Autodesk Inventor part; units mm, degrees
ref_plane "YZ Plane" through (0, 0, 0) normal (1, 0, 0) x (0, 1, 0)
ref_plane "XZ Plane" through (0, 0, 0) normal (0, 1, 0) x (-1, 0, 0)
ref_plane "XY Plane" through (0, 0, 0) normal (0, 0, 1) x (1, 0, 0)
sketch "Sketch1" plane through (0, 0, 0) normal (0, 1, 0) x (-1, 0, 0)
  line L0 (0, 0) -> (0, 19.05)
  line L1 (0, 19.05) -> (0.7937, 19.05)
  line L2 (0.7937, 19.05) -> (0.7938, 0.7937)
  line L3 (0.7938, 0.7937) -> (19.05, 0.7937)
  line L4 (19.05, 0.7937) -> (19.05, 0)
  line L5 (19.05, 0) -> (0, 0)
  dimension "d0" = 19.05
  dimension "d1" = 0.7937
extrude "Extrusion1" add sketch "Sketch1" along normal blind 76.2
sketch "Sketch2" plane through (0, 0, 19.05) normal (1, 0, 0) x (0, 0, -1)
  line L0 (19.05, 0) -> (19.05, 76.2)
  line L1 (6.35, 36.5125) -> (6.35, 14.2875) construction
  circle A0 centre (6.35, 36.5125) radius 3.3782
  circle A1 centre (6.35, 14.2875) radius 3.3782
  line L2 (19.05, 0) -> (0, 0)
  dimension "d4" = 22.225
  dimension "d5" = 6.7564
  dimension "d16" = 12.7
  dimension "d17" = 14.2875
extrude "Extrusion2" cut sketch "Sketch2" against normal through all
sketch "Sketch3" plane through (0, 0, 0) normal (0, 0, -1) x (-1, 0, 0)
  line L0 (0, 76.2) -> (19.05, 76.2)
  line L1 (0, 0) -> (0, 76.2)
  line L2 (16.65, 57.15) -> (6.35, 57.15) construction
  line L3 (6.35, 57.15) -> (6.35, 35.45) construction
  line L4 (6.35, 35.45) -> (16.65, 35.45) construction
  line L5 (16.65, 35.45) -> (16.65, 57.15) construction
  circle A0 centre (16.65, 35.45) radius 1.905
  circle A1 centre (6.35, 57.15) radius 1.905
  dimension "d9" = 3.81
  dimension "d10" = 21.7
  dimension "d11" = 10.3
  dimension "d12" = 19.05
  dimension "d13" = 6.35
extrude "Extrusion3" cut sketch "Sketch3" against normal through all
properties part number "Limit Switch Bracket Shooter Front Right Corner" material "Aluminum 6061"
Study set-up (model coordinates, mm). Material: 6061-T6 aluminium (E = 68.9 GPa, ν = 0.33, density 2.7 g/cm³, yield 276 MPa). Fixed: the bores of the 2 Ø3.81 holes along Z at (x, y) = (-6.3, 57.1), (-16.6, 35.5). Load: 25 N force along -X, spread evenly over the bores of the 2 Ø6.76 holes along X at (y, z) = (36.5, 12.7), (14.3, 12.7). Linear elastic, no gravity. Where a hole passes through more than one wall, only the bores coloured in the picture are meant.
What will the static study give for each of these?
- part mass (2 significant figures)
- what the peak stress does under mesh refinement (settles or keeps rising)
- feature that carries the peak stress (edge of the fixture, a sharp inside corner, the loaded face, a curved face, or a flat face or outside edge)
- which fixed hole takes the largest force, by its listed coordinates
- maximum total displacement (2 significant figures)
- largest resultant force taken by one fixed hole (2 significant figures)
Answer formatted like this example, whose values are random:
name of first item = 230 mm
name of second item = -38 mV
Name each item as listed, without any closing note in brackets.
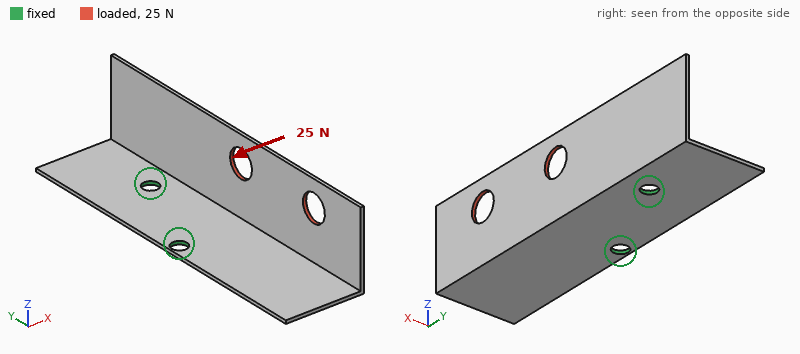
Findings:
part mass = 5.9 g
what the peak stress does under mesh refinement = keeps rising
feature that carries the peak stress = edge of the fixture
which fixed hole takes the largest force, by its listed coordinates = (-16.6, 35.5)
maximum total displacement = 0.93 mm
largest resultant force taken by one fixed hole = 32 N
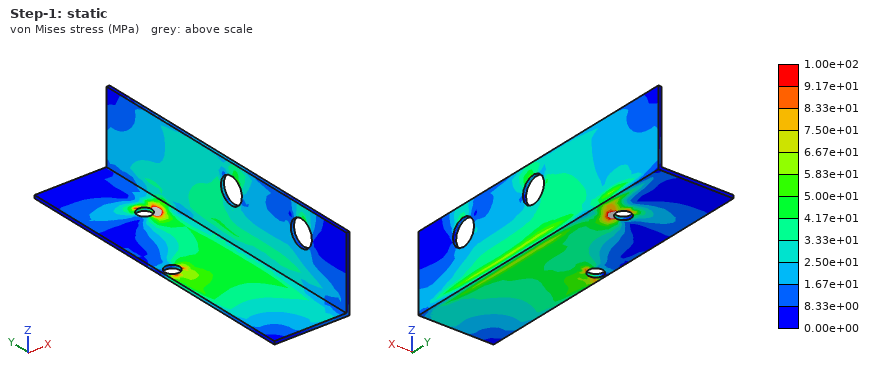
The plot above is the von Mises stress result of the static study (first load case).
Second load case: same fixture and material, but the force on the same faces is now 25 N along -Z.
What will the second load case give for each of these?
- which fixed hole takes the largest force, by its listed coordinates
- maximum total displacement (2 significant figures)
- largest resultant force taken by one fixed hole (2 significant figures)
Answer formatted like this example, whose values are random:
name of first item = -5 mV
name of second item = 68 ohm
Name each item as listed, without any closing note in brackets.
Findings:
which fixed hole takes the largest force, by its listed coordinates = (-16.6, 35.5)
maximum total displacement = 0.82 mm
largest resultant force taken by one fixed hole = 20 N
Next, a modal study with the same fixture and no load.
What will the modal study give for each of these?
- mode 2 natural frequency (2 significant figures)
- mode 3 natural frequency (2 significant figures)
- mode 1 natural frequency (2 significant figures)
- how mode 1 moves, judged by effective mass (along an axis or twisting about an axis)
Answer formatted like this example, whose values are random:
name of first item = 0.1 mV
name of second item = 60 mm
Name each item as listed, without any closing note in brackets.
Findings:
mode 2 natural frequency = 1000 Hz
mode 3 natural frequency = 1400 Hz
mode 1 natural frequency = 630 Hz
how mode 1 moves, judged by effective mass = along Z
